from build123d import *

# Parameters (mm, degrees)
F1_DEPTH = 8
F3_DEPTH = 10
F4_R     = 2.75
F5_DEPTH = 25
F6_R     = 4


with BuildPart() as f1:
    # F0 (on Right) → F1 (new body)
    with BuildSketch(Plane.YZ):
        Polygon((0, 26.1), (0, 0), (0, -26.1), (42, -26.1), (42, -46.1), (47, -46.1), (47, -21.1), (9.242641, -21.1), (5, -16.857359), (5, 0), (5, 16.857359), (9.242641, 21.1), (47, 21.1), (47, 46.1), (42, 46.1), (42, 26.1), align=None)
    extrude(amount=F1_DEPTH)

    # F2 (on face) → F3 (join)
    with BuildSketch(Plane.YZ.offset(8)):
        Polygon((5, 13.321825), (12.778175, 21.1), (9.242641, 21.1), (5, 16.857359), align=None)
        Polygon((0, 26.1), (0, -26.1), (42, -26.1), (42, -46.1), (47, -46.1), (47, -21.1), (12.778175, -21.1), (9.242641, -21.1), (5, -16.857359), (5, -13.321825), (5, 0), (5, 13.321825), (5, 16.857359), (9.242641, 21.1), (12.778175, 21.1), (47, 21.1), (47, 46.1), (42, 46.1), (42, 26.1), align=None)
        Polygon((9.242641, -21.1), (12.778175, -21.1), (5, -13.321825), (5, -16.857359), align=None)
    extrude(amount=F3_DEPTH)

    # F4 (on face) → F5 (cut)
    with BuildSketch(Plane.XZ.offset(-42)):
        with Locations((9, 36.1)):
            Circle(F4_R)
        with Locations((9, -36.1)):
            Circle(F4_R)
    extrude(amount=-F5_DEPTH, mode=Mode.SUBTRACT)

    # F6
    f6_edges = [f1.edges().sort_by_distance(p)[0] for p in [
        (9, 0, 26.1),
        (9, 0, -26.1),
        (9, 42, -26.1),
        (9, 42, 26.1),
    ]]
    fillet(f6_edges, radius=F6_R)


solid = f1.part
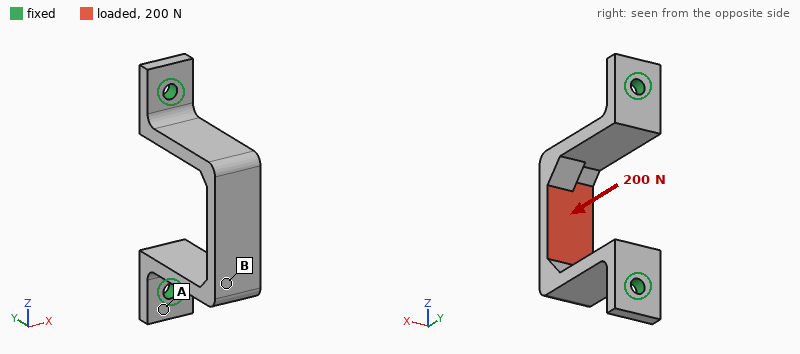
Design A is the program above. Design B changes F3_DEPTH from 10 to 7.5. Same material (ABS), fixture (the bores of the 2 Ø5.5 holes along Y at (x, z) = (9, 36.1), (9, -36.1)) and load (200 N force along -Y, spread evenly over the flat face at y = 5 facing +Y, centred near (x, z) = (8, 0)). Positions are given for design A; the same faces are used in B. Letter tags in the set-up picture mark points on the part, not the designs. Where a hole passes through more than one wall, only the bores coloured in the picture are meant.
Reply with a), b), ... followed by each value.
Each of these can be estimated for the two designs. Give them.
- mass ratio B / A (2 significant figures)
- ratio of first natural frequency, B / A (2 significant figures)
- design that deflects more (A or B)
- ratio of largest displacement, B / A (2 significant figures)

a) 0.86
b) 0.97
c) B
d) 1.2
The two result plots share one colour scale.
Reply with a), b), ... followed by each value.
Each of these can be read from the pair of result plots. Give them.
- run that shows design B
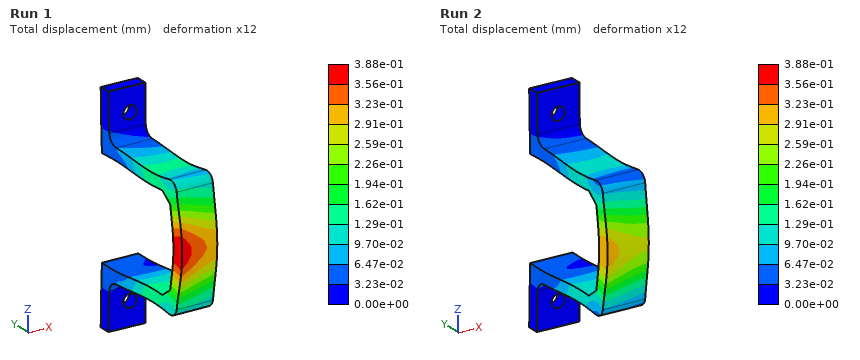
a) Run 1
